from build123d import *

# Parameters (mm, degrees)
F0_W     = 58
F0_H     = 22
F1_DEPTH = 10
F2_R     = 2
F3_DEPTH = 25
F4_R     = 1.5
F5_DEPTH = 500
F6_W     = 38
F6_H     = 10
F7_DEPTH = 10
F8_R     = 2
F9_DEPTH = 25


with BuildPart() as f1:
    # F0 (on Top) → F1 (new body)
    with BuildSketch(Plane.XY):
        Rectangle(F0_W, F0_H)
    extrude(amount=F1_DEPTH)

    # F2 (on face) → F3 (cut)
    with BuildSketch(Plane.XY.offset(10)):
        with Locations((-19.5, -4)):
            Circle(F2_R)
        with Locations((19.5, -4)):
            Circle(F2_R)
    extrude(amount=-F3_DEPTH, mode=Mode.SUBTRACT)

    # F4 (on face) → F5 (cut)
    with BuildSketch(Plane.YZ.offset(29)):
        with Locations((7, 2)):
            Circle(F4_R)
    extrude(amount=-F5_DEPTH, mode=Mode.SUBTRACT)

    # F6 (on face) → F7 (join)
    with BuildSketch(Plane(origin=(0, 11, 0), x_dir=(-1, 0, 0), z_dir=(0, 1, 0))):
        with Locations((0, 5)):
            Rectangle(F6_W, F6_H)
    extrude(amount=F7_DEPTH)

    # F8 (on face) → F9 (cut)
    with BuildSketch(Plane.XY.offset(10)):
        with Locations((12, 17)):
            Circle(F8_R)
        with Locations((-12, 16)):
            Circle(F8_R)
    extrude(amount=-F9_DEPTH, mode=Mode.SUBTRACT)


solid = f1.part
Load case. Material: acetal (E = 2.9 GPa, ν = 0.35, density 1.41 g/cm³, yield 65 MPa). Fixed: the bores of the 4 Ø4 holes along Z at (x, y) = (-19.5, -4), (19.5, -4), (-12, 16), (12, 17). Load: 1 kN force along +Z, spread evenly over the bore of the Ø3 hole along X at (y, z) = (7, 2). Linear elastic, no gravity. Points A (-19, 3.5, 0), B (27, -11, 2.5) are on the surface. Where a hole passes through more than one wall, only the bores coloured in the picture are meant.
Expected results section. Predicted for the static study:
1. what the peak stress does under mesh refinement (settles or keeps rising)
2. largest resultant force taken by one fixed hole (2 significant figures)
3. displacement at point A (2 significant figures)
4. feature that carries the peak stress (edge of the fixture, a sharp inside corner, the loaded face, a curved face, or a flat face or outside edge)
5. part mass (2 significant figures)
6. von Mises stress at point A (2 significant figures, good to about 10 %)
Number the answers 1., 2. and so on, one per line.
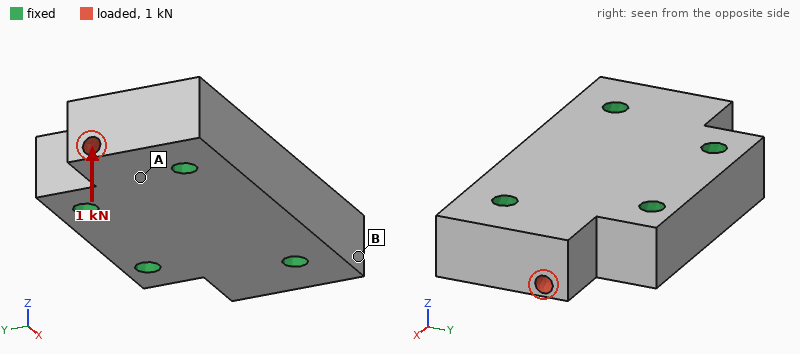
1. keeps rising
2. 270 N
3. 18 µm
4. edge of the fixture
5. 22 g
6. 2.6 MPa
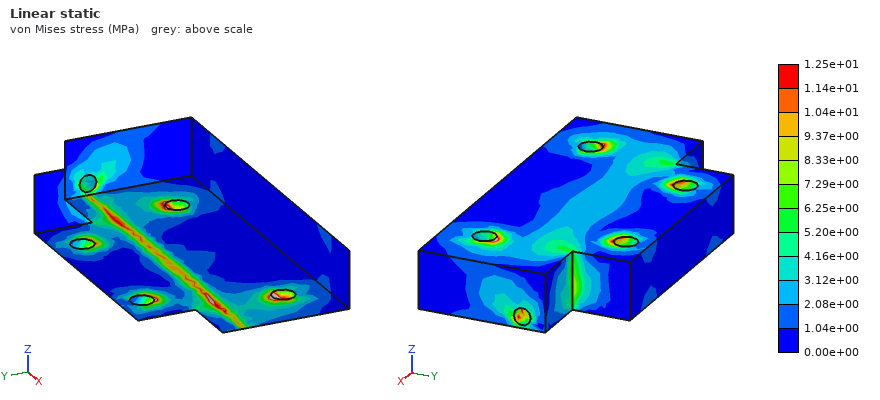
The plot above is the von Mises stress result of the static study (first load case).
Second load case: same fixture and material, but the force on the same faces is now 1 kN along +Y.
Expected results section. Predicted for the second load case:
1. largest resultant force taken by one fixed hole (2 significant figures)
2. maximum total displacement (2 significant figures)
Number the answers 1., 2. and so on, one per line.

1. 260 N
2. 26 µm
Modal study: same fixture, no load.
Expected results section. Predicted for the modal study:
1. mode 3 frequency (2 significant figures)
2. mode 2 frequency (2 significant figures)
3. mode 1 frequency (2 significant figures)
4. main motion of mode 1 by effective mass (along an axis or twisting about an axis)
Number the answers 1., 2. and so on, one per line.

1. 11 kHz
2. 11 kHz
3. 7600 Hz
4. along Z
